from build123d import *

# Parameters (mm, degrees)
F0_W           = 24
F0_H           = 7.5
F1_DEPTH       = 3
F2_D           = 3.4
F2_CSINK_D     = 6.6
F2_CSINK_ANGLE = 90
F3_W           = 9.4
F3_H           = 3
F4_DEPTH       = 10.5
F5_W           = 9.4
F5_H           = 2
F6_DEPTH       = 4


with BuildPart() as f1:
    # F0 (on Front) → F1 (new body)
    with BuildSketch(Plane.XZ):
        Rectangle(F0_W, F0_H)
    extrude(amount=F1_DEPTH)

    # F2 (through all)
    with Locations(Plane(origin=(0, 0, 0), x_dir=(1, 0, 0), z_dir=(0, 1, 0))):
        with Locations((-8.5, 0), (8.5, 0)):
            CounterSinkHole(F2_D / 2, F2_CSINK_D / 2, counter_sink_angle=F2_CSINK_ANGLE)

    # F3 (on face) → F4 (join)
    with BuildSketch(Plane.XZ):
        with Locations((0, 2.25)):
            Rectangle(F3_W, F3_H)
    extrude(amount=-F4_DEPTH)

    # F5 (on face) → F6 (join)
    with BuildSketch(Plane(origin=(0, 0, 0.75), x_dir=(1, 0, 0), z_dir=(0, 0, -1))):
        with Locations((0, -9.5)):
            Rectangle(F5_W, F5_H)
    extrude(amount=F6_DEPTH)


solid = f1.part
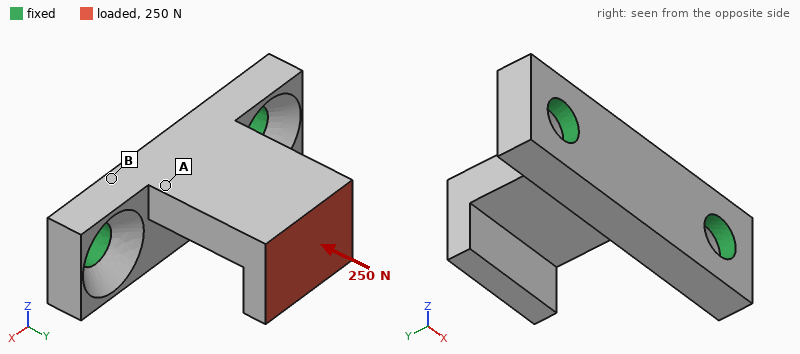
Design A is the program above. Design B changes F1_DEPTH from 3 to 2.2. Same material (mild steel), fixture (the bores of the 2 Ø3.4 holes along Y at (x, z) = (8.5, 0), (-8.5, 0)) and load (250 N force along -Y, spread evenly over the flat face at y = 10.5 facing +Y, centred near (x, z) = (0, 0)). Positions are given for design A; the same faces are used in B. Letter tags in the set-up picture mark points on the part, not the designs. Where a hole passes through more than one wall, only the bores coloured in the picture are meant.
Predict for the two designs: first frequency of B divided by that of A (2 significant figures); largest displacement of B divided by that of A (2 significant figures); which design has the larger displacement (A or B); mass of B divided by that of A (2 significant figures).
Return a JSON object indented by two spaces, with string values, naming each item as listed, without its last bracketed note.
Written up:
{
  "first frequency of B divided by that of A": "0.72",
  "largest displacement of B divided by that of A": "1.1",
  "which design has the larger displacement": "B",
  "mass of B divided by that of A": "0.84"
}
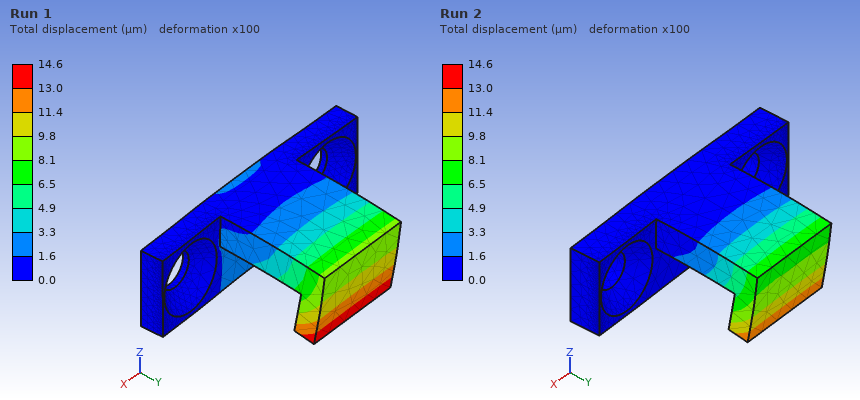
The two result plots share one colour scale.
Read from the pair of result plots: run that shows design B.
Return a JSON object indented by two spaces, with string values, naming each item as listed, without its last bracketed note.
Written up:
{
  "run that shows design B": "Run 1"
}
